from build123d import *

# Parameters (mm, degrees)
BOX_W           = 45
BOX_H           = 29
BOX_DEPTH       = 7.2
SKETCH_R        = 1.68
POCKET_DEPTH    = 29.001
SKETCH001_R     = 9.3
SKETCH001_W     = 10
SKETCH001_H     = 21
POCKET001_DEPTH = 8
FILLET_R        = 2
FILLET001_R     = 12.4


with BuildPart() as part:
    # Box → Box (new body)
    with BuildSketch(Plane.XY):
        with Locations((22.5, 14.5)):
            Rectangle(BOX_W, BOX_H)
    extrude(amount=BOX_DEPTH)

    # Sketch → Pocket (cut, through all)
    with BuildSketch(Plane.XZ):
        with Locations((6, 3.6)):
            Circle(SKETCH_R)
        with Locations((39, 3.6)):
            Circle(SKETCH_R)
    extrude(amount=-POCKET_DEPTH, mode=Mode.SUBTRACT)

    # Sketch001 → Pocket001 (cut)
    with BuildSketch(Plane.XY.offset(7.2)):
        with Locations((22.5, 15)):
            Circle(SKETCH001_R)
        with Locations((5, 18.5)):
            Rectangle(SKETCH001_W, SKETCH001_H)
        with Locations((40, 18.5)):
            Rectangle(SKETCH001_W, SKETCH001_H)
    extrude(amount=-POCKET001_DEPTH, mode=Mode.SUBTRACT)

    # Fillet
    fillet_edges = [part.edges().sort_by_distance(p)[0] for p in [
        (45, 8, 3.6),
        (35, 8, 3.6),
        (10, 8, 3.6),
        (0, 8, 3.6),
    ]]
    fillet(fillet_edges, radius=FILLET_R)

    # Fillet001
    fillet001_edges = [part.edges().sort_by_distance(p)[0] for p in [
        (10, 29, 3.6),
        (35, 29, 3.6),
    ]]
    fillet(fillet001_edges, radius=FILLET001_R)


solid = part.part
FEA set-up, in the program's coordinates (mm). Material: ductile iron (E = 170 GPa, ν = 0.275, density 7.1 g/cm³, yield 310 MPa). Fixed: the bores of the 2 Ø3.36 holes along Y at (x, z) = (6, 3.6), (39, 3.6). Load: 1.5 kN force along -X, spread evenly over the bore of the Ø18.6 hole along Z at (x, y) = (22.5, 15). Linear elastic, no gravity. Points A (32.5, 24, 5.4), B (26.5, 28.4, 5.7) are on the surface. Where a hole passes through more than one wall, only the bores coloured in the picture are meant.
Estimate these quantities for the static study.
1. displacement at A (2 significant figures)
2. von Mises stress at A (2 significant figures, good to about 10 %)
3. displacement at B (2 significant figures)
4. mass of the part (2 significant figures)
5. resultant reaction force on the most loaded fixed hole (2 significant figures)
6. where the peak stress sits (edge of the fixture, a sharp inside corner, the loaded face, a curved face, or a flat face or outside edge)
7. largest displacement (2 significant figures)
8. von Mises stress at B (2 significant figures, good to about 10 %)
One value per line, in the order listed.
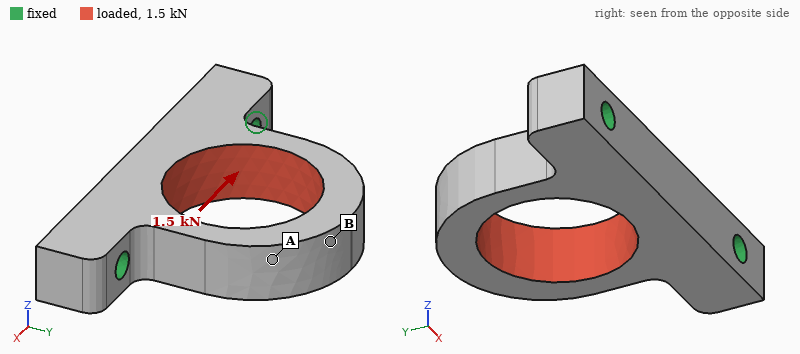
23 µm
53 MPa
22 µm
27 g
880 N
a curved face
23 µm
22 MPa
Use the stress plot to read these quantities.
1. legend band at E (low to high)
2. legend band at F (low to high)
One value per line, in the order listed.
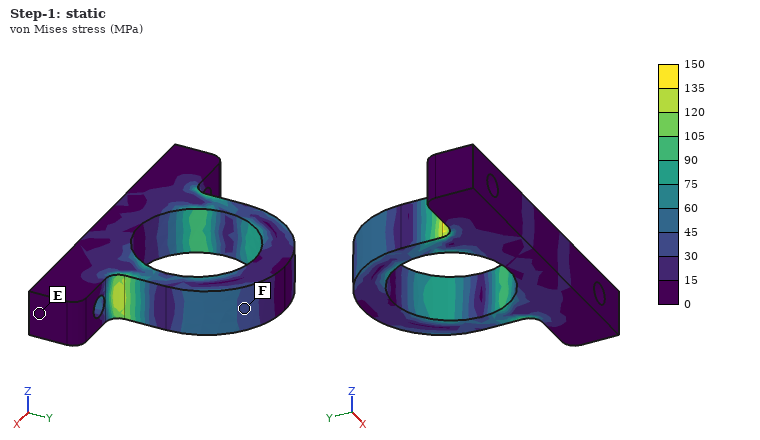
0 to 15 MPa
30 to 45 MPa
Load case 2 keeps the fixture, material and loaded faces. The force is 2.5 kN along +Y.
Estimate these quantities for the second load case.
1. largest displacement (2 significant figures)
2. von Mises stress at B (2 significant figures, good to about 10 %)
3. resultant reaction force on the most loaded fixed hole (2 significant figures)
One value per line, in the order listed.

6.9 µm
19 MPa
1.3 kN
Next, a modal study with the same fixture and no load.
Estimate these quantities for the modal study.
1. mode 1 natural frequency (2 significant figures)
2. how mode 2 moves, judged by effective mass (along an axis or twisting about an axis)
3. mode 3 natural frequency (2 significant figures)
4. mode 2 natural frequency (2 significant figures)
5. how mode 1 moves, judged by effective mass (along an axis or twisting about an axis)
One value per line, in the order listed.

6600 Hz
along X
17 kHz
11 kHz
along Z
